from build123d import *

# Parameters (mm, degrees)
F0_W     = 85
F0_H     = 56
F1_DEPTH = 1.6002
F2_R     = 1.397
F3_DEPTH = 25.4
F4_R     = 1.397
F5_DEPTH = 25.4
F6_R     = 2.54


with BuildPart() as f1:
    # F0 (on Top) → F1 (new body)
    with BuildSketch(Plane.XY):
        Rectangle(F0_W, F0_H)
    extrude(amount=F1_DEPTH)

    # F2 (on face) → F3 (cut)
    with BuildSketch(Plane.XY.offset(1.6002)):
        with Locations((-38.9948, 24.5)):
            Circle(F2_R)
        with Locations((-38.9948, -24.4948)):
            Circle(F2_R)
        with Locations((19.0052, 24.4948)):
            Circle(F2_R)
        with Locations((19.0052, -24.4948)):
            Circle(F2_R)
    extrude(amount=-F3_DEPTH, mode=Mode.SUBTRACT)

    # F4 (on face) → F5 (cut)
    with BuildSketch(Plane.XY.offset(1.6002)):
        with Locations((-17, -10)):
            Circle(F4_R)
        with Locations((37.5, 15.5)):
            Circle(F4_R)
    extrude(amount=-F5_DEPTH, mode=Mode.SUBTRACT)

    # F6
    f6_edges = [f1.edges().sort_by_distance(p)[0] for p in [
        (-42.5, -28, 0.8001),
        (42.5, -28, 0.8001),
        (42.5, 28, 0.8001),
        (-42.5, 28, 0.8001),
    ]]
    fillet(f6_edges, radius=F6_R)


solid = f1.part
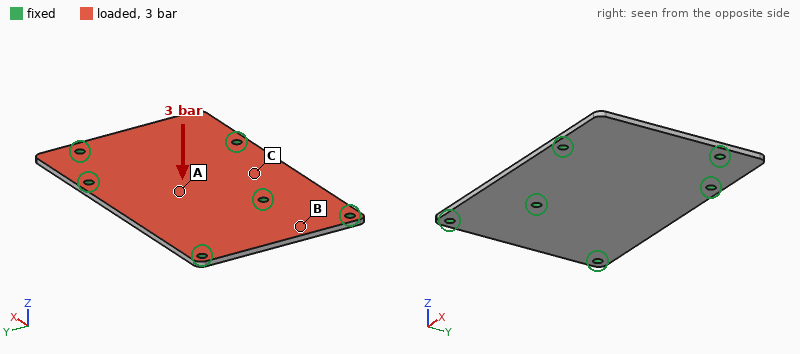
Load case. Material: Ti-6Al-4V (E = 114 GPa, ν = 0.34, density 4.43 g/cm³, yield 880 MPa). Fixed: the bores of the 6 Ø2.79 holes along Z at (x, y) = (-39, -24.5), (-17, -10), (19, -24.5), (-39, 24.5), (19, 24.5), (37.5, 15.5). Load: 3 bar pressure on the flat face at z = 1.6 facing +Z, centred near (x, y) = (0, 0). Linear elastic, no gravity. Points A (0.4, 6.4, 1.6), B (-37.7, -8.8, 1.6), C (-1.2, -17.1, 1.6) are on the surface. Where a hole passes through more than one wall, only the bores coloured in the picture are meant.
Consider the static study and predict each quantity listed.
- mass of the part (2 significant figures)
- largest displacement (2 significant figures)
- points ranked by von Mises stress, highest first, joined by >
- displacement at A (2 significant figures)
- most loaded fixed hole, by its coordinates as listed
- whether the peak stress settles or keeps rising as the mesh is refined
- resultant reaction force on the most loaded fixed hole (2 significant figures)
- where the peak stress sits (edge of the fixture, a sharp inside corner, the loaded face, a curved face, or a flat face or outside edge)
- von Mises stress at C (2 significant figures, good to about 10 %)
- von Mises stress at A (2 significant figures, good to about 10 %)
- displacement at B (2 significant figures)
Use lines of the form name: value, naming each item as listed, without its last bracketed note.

mass of the part: 33 g
largest displacement: 0.21 mm
points ranked by von Mises stress, highest first, joined by >: A > C > B
displacement at A: 0.14 mm
most loaded fixed hole, by its coordinates as listed: (-17, -10)
whether the peak stress settles or keeps rising as the mesh is refined: keeps rising
resultant reaction force on the most loaded fixed hole: 420 N
where the peak stress sits: edge of the fixture
von Mises stress at C: 52 MPa
von Mises stress at A: 67 MPa
displacement at B: 0.043 mm
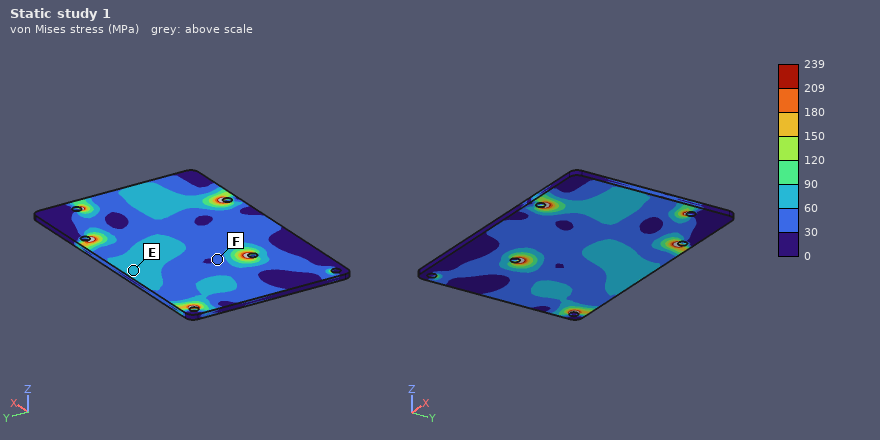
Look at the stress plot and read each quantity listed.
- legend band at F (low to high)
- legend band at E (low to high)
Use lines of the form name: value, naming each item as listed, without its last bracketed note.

legend band at F: 30 to 60 MPa
legend band at E: 60 to 90 MPa
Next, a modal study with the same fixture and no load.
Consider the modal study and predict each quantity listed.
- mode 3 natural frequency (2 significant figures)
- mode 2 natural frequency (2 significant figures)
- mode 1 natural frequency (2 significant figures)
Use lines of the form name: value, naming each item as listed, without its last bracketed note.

mode 3 natural frequency: 4100 Hz
mode 2 natural frequency: 2900 Hz
mode 1 natural frequency: 2800 Hz
